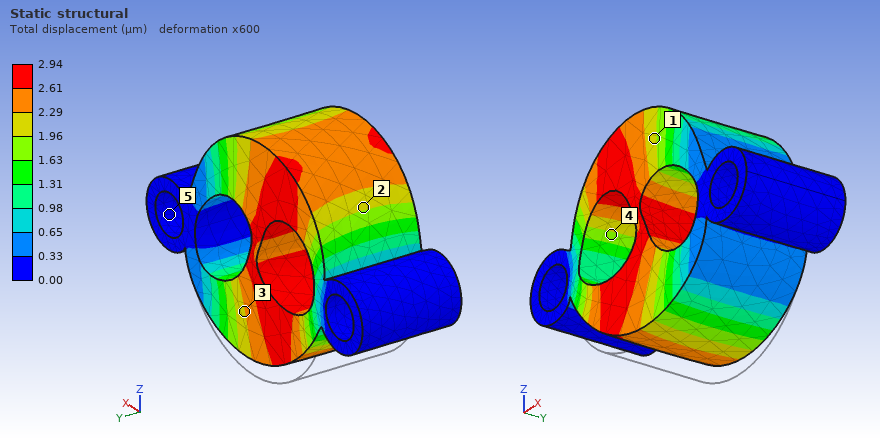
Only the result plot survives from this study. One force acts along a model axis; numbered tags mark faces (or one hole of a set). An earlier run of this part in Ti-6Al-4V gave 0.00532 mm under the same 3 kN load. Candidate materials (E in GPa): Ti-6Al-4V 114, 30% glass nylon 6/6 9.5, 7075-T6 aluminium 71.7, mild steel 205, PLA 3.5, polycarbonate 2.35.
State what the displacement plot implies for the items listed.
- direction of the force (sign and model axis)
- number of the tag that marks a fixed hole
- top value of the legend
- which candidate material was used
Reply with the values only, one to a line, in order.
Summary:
+Z
5
2.94 µm
mild steel
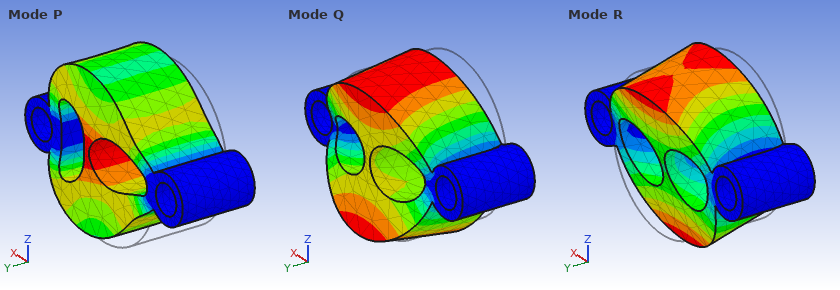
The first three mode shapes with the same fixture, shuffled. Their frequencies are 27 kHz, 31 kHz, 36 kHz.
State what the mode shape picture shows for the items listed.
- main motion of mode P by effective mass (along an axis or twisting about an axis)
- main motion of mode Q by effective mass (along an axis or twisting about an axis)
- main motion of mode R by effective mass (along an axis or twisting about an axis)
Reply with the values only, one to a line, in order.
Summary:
along X
along Y
twisting about X
